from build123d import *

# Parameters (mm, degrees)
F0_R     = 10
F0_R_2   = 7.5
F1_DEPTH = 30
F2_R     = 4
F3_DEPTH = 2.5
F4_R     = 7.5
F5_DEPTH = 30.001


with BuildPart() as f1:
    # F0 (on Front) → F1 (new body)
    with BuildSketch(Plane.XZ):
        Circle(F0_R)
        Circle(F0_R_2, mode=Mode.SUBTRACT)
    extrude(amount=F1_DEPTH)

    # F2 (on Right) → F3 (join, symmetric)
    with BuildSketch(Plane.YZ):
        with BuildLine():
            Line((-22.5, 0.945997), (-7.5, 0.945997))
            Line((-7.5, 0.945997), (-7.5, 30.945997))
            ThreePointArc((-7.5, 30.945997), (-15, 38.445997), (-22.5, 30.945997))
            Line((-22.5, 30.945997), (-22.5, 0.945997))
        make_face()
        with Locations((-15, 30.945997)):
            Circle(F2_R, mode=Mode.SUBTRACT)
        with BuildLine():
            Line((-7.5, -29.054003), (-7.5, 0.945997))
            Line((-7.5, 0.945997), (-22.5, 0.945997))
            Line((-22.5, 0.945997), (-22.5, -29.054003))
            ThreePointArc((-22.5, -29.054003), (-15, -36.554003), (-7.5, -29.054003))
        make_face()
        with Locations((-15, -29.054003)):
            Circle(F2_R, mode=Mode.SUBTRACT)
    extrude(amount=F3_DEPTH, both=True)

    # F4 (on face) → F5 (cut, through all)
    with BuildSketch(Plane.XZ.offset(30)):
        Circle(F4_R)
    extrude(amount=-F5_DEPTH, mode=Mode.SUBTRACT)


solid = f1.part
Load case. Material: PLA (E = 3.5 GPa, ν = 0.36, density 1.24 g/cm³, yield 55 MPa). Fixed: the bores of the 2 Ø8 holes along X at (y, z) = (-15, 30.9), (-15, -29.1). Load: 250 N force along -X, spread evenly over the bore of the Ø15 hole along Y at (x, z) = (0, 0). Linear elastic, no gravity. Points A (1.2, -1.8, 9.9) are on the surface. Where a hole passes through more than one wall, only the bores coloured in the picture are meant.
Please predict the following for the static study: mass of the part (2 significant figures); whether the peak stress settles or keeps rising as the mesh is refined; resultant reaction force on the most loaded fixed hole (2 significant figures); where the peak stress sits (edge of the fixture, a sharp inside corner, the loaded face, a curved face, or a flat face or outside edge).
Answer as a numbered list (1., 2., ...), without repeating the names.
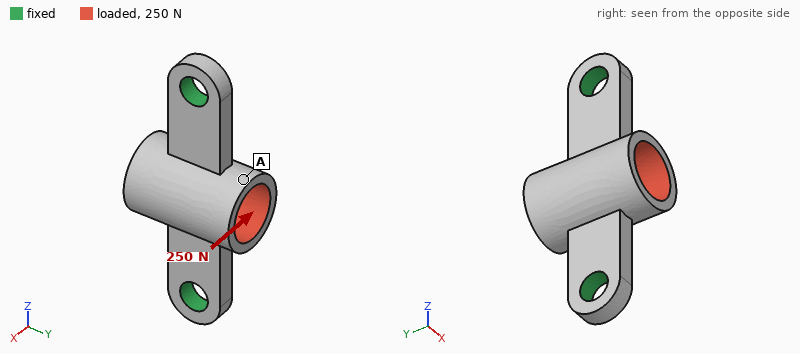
1. 9.3 g
2. keeps rising
3. 130 N
4. edge of the fixture
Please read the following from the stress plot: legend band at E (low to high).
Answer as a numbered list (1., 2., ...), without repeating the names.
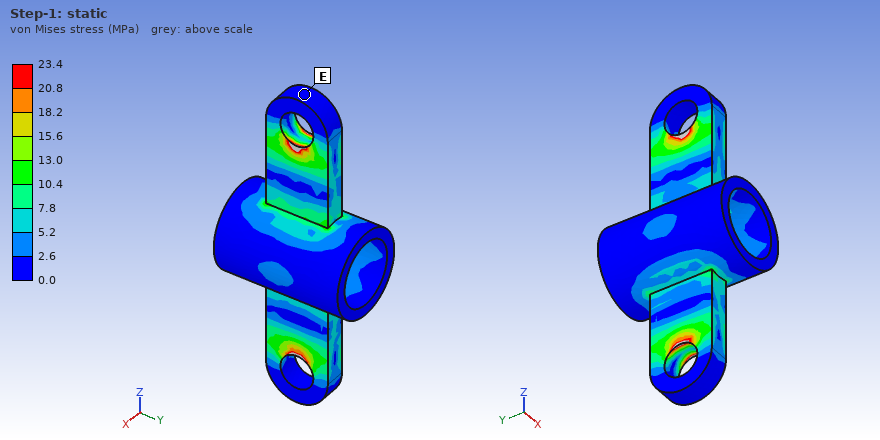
1. 0.0 to 2.6 MPa
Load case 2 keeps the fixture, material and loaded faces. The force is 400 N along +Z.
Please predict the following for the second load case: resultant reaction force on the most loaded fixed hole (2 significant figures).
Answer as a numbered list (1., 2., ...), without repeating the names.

1. 200 N
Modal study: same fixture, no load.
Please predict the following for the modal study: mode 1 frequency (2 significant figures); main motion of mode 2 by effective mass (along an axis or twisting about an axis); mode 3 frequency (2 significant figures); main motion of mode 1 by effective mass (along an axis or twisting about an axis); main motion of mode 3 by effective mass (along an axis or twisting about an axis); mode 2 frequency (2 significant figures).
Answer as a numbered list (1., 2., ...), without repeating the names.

1. 1900 Hz
2. along X
3. 3400 Hz
4. twisting about Z
5. along Y
6. 2300 Hz
